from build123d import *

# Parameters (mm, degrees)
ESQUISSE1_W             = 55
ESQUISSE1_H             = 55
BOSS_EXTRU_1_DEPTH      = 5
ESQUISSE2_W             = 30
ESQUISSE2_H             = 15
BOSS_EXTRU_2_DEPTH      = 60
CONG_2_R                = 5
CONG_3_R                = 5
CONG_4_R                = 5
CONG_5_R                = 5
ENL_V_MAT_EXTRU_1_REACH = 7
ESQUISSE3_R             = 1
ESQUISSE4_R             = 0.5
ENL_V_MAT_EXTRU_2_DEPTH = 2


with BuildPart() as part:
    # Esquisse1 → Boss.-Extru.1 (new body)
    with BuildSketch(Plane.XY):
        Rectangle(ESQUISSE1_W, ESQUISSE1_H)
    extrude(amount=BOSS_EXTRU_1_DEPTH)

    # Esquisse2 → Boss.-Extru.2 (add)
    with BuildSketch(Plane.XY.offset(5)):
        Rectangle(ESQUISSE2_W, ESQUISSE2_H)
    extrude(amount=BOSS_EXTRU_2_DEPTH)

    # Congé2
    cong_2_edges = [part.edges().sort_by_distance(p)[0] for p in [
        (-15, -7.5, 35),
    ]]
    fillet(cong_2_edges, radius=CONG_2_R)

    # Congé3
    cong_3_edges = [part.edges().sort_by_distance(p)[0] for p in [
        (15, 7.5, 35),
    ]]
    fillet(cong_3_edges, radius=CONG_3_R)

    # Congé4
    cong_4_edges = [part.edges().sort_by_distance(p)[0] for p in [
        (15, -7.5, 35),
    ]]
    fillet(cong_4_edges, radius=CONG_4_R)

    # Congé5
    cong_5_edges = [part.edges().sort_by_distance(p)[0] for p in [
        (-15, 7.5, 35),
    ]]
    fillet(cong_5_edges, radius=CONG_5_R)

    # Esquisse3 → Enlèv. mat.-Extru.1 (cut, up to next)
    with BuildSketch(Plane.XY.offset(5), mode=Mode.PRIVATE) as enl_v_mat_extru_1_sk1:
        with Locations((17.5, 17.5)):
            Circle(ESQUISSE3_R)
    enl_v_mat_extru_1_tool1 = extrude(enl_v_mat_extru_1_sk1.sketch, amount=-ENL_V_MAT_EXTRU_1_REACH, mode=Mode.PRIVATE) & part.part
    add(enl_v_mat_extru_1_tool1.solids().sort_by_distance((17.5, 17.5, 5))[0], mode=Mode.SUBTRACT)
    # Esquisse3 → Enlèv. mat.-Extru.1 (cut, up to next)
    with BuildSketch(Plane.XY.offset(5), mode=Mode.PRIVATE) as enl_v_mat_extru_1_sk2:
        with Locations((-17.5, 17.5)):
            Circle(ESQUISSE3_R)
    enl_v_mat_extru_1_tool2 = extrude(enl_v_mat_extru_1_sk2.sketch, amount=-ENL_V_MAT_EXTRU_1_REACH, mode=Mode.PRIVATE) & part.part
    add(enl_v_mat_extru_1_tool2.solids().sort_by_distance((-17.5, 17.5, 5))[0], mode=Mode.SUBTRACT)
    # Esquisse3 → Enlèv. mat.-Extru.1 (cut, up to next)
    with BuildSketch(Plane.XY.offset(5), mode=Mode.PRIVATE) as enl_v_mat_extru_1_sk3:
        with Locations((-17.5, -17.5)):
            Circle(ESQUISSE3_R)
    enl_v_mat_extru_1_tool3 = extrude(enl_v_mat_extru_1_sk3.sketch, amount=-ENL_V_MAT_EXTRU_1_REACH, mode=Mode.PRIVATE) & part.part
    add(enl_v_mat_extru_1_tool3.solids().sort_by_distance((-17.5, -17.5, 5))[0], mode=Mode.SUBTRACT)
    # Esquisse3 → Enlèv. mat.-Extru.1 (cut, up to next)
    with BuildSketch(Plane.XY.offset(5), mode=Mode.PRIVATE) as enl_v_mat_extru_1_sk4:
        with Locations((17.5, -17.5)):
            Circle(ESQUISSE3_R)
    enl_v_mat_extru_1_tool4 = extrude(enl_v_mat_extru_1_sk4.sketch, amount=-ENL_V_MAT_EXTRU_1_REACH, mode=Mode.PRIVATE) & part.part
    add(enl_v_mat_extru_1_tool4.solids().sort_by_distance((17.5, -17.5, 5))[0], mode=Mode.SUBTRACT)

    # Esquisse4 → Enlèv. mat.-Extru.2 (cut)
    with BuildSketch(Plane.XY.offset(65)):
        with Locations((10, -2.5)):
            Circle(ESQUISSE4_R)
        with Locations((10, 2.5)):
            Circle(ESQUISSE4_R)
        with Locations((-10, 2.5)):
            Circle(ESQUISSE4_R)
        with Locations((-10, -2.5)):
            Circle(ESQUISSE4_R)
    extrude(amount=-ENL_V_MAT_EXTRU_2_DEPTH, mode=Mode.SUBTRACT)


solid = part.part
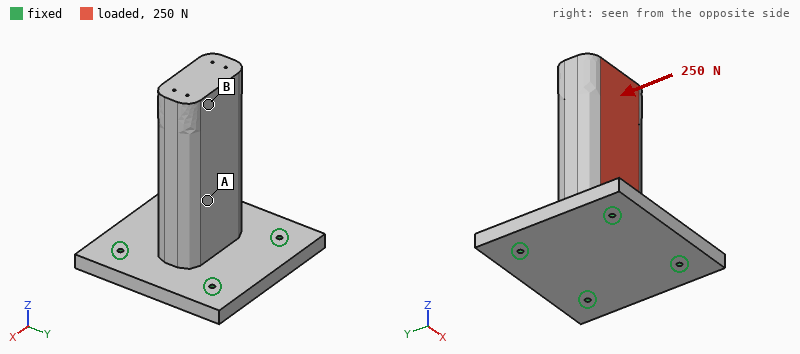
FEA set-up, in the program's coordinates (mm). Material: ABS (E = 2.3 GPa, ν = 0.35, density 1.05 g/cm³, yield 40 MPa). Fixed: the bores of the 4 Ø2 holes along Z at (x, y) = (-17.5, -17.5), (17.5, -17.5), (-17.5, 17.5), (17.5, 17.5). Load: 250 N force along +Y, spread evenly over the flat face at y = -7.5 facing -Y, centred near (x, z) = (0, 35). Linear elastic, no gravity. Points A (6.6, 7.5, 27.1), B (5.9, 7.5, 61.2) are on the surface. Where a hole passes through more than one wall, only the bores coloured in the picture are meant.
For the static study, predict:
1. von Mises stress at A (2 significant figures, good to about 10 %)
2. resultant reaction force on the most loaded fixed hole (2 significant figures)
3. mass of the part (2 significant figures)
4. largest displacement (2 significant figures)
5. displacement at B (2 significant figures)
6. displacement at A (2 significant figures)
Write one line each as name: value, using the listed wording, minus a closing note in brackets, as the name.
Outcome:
von Mises stress at A: 3.0 MPa
resultant reaction force on the most loaded fixed hole: 150 N
mass of the part: 43 g
largest displacement: 1.1 mm
displacement at B: 1.0 mm
displacement at A: 0.38 mm
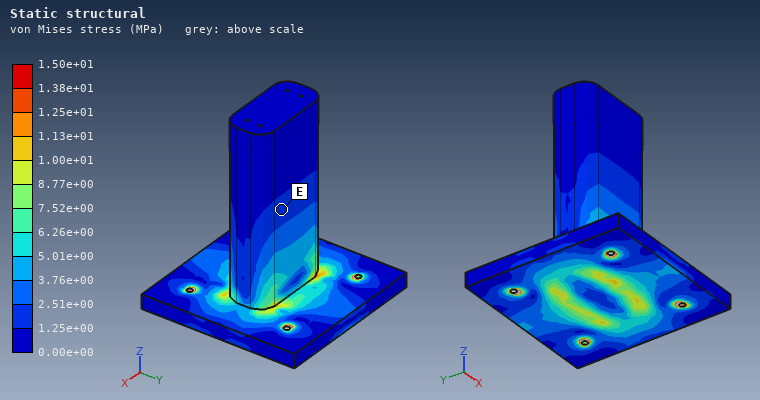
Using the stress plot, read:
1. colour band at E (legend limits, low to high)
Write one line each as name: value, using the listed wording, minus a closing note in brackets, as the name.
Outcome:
colour band at E: 1.25e+00 to 2.51e+00 MPa
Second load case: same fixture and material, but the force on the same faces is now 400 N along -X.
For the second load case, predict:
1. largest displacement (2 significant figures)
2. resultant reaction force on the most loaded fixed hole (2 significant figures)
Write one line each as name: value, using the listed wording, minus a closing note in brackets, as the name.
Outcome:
largest displacement: 0.99 mm
resultant reaction force on the most loaded fixed hole: 220 N
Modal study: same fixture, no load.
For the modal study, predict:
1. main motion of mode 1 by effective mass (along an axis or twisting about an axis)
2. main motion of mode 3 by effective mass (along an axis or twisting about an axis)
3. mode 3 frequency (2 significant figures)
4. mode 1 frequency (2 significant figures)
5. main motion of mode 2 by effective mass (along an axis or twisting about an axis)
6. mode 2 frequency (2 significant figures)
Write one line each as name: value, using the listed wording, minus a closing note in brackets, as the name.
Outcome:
main motion of mode 1 by effective mass: along Y
main motion of mode 3 by effective mass: along Z
mode 3 frequency: 1700 Hz
mode 1 frequency: 570 Hz
main motion of mode 2 by effective mass: along X
mode 2 frequency: 750 Hz
